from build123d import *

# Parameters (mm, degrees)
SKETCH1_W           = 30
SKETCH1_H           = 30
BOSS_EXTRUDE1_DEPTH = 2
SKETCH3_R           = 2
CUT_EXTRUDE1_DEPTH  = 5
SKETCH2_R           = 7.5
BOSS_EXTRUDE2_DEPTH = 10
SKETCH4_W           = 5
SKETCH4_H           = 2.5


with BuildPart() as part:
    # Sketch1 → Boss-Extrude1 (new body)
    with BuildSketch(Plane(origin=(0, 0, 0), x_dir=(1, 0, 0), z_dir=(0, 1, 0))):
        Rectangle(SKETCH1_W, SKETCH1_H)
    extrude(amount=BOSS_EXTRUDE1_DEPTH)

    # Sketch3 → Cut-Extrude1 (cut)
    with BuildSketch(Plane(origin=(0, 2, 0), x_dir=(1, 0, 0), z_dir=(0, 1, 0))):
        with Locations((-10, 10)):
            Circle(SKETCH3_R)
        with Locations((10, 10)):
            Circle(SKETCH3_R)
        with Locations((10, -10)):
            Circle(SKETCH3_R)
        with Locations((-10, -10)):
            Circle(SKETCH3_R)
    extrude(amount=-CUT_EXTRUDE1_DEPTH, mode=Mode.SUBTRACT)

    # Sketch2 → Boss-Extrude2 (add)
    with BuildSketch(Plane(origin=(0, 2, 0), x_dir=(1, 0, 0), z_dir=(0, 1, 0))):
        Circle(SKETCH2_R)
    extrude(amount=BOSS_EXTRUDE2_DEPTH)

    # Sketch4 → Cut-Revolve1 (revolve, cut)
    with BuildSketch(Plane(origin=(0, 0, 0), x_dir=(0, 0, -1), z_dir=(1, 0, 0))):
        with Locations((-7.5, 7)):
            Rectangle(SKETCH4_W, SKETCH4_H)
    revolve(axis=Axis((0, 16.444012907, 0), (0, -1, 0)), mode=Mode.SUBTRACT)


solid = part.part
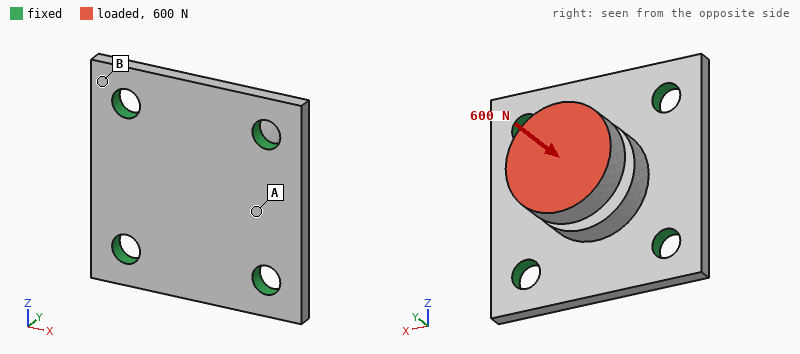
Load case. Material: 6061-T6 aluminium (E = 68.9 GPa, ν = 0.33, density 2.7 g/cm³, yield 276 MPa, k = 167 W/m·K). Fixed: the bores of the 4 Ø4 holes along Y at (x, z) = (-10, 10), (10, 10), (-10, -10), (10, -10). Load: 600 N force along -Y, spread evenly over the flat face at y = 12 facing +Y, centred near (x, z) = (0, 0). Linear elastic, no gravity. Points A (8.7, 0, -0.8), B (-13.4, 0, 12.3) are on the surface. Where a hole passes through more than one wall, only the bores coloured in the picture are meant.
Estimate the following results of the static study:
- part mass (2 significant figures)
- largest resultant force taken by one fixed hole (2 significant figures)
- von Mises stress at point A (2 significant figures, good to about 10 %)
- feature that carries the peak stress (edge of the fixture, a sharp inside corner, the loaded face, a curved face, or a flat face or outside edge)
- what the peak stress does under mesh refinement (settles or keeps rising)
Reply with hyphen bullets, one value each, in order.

- 8.7 g
- 160 N
- 20 MPa
- edge of the fixture
- keeps rising
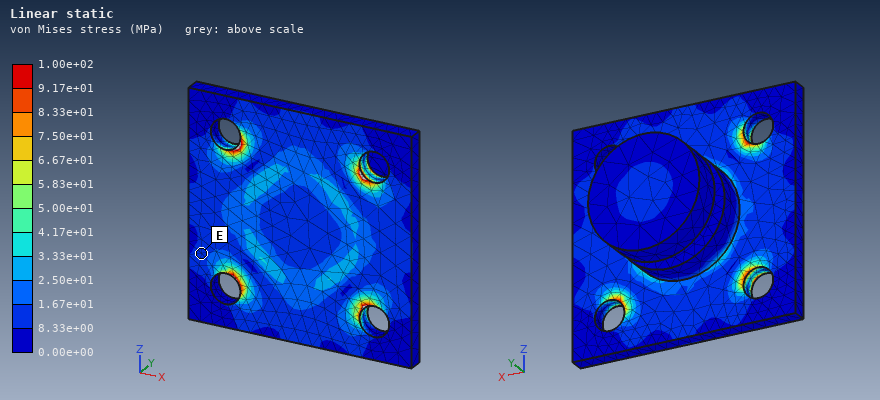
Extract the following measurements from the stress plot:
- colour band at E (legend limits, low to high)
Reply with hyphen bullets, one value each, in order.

- 8.33e+00 to 1.67e+01 MPa
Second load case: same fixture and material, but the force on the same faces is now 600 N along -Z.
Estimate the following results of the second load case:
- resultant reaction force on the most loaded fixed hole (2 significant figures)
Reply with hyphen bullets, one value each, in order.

- 270 N
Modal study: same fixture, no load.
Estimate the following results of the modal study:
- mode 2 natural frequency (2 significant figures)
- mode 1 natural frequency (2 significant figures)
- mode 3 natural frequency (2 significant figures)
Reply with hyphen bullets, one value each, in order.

- 17 kHz
- 17 kHz
- 17 kHz
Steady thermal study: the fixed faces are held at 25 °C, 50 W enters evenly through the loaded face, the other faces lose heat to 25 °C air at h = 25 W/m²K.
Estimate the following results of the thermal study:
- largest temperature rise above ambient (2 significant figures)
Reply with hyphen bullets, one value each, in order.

- 53 K
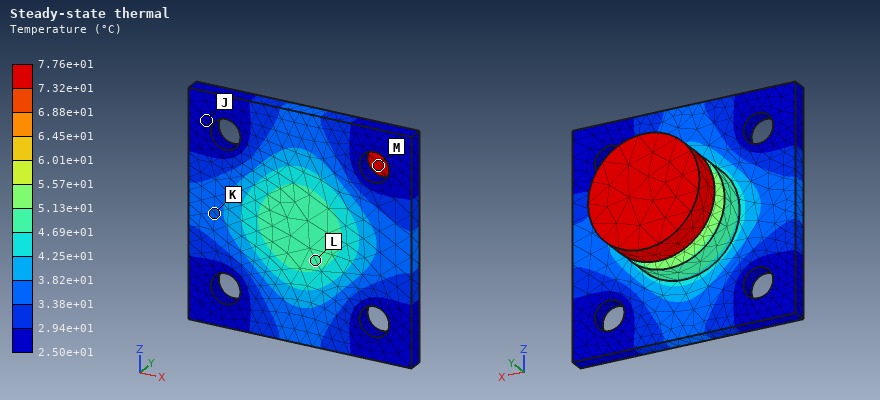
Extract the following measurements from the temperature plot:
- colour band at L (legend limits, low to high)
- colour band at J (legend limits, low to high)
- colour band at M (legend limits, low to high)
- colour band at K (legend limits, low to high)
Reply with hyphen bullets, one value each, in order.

- 4.69e+01 to 5.13e+01 °C
- 2.50e+01 to 2.94e+01 °C
- 7.32e+01 to 7.76e+01 °C
- 3.38e+01 to 3.82e+01 °C
